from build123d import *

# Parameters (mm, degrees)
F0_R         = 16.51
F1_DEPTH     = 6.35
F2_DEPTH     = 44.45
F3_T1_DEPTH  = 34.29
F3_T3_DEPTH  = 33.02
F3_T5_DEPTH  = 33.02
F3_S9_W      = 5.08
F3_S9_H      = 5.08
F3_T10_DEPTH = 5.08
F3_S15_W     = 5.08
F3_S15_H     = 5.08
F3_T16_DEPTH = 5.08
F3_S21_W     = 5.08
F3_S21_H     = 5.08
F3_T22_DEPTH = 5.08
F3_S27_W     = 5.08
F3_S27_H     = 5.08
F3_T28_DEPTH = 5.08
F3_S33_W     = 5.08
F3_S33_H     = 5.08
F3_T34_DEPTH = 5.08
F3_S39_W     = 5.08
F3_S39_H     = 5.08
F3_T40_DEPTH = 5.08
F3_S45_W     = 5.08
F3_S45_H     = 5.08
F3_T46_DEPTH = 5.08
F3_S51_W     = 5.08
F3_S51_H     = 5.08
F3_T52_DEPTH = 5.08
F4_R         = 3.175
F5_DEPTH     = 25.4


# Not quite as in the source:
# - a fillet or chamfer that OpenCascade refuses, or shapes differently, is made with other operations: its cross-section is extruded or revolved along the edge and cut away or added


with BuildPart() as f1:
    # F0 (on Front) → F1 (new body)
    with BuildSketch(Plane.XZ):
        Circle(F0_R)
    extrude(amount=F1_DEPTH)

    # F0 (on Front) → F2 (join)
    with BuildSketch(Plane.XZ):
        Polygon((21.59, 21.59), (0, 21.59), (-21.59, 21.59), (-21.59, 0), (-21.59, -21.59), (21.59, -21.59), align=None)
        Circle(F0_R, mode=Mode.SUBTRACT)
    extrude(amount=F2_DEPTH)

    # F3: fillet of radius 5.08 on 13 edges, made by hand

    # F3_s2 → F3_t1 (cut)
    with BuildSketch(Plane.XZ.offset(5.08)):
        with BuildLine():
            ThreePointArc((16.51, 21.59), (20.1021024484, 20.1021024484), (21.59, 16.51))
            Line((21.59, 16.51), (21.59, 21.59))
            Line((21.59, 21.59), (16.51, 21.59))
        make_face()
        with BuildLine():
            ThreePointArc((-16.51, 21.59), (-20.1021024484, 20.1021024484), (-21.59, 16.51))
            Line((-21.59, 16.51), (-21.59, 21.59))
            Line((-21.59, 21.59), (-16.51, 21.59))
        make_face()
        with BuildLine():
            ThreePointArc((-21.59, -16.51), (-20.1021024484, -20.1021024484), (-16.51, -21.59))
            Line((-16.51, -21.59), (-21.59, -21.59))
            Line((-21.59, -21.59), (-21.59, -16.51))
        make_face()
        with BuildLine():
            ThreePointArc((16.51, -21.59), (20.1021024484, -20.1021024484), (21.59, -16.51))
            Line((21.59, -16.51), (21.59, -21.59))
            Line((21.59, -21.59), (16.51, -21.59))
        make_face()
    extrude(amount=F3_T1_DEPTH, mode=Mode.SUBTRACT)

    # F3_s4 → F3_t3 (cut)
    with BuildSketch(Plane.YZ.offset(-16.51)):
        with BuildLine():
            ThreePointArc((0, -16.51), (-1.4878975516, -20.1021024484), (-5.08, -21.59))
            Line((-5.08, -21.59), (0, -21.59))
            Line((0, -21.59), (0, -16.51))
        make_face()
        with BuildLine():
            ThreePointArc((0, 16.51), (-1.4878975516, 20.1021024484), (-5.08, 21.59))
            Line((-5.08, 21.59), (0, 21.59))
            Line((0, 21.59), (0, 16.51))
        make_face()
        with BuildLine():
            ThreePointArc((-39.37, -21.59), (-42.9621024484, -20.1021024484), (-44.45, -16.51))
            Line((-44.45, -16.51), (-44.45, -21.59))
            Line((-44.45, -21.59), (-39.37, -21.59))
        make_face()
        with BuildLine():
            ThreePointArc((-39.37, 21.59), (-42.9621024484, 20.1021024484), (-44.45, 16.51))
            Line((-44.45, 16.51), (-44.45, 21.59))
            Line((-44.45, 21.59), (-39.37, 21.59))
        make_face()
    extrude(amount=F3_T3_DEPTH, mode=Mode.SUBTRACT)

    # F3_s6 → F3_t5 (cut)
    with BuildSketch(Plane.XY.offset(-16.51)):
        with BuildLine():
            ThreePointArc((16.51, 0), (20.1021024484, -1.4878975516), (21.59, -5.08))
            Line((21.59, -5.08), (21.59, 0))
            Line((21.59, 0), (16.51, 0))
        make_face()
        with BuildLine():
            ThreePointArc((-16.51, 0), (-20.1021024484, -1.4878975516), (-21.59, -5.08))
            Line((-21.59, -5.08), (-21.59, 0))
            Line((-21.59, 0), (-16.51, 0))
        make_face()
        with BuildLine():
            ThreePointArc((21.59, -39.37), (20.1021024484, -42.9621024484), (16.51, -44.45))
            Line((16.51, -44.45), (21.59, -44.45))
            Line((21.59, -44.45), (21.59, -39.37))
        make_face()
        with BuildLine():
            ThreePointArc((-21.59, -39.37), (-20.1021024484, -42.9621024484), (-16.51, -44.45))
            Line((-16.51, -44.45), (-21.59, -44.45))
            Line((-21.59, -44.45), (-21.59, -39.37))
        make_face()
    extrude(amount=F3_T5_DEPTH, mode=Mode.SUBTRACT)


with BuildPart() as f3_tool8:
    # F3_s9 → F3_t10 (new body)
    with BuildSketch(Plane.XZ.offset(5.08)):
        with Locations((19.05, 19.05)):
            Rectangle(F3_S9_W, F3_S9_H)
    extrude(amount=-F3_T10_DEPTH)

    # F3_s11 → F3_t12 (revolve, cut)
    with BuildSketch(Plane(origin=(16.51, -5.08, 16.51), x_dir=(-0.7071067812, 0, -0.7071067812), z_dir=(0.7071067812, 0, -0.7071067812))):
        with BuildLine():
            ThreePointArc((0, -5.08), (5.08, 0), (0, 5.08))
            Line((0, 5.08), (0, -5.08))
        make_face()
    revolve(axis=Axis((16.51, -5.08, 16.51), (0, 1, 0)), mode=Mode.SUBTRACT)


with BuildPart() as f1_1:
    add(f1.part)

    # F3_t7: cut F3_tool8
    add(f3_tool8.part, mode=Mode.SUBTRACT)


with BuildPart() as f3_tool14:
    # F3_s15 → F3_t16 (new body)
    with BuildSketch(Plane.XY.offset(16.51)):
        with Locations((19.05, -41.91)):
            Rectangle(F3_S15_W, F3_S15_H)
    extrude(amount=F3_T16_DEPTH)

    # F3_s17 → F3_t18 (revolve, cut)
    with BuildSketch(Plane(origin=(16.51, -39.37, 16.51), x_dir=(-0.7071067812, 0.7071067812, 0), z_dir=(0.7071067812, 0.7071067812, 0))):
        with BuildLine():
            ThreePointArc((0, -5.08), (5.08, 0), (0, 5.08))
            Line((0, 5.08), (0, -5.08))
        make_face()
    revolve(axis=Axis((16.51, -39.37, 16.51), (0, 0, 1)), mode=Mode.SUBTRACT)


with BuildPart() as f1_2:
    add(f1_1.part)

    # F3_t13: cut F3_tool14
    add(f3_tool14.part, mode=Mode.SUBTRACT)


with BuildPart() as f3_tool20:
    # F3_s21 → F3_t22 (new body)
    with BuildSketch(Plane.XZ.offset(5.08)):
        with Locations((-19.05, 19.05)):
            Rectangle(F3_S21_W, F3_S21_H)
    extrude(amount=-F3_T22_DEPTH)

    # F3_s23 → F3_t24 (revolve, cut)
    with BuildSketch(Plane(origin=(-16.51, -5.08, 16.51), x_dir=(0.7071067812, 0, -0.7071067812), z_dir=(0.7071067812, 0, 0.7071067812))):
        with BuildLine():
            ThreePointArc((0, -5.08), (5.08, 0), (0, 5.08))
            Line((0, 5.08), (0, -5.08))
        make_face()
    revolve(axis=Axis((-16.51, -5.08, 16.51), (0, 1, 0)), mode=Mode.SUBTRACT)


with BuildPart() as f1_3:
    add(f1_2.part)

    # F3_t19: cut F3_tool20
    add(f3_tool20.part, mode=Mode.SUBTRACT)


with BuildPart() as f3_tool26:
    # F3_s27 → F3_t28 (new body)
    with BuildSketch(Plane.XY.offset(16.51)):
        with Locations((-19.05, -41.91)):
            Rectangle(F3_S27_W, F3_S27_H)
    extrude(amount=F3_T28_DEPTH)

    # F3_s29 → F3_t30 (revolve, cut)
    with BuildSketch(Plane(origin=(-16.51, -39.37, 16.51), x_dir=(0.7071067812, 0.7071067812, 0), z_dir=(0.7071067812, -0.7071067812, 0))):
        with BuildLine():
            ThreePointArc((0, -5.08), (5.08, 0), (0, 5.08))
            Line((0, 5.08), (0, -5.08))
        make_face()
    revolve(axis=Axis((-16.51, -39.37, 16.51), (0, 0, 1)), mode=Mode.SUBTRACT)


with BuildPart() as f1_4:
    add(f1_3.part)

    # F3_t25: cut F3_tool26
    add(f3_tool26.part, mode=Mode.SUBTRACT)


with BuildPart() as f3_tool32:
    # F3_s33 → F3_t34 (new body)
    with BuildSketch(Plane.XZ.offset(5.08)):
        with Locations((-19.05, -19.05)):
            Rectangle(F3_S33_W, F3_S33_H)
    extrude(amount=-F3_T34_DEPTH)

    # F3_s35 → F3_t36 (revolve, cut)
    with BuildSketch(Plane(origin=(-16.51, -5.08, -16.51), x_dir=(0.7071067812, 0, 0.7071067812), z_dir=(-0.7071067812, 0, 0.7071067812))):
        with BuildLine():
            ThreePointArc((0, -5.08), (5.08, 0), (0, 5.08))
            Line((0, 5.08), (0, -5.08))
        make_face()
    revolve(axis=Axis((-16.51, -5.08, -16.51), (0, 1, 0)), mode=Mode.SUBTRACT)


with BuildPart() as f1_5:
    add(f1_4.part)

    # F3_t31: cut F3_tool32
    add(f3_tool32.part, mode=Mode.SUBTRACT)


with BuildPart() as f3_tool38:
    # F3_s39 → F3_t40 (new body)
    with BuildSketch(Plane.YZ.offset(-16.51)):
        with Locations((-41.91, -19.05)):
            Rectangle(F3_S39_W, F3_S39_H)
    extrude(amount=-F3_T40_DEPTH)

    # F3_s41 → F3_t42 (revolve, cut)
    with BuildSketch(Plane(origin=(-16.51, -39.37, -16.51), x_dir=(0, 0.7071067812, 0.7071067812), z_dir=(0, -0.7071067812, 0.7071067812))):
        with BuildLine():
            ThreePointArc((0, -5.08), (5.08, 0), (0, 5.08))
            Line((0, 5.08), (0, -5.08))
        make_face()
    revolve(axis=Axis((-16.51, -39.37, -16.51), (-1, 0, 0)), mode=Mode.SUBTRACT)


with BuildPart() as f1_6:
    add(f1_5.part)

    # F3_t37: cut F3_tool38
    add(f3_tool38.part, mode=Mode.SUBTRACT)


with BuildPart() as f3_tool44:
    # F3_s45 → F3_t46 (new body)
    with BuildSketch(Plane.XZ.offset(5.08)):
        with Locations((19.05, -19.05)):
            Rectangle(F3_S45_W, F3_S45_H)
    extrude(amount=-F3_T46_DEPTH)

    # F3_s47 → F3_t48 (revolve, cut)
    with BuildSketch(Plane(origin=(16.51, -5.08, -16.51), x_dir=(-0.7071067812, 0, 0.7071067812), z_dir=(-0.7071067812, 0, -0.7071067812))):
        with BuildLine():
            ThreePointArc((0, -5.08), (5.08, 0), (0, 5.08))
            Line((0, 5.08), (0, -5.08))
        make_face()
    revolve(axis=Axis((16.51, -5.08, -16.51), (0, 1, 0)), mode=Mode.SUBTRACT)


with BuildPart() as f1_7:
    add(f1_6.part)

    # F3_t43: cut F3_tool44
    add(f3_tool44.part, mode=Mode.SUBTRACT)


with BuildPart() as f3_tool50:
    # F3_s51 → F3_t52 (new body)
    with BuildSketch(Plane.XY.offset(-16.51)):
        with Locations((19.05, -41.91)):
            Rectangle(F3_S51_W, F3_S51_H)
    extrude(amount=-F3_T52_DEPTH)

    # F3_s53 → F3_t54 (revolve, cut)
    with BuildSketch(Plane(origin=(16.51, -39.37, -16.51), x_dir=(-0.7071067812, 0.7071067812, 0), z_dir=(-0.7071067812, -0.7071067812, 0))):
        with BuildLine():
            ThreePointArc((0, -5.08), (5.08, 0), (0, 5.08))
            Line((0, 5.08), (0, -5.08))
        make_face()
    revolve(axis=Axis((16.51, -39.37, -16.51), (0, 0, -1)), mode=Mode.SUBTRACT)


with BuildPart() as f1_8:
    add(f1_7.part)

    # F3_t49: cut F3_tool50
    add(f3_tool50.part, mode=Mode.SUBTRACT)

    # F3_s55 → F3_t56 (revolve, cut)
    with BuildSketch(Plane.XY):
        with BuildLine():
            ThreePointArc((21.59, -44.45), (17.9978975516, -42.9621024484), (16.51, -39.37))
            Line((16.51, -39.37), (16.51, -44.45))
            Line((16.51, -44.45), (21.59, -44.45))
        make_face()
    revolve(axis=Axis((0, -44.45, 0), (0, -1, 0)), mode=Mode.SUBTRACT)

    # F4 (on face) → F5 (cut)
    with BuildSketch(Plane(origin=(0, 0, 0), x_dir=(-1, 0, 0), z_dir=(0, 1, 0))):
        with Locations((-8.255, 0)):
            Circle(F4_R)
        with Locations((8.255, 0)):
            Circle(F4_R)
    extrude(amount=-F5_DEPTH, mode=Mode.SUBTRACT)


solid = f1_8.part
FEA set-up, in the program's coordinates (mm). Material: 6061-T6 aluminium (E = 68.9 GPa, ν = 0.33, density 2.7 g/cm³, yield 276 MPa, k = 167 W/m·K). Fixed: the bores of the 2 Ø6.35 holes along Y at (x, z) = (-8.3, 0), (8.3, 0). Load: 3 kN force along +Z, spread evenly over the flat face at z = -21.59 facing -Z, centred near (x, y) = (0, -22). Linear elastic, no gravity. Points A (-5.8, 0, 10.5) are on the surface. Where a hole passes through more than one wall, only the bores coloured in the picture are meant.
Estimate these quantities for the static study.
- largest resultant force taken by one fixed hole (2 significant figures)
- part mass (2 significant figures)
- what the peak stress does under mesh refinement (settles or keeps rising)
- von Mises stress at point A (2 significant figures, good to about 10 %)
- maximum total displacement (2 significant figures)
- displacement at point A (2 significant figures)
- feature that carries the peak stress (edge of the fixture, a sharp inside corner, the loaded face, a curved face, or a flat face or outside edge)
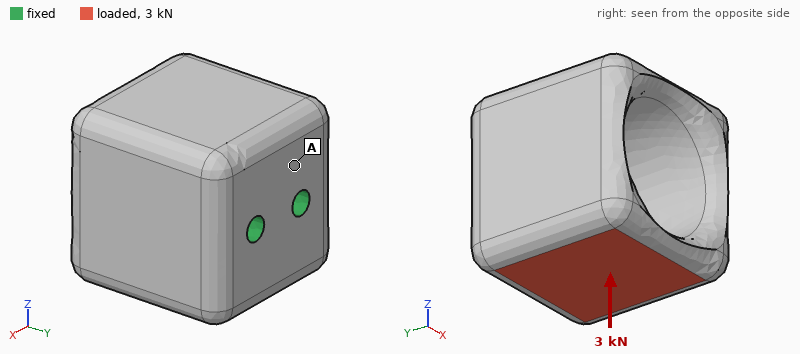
1.5 kN
130 g
keeps rising
27 MPa
0.13 mm
0.020 mm
edge of the fixture
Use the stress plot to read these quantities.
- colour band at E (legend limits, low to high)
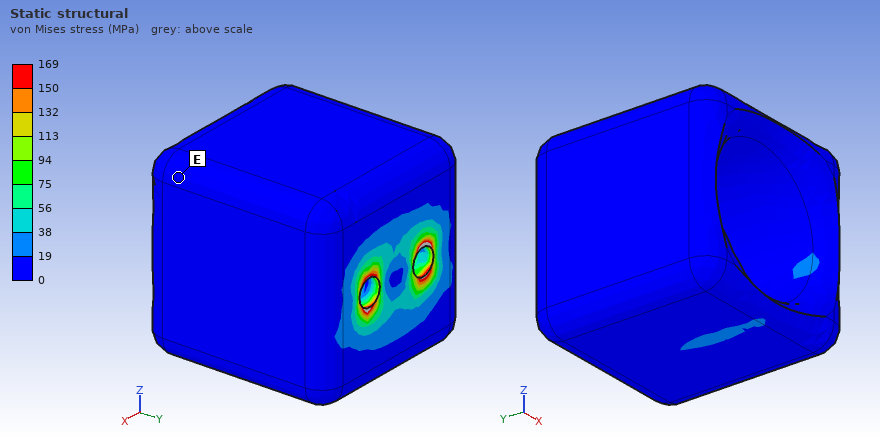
0 to 19 MPa
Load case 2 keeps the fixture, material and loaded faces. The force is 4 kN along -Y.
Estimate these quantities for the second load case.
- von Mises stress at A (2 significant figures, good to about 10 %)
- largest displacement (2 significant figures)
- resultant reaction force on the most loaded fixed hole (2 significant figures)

34 MPa
0.17 mm
2.0 kN
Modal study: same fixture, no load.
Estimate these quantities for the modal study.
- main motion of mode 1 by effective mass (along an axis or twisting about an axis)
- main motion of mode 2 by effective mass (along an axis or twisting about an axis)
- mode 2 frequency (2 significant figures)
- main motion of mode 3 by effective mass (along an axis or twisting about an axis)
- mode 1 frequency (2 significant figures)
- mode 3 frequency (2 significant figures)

along Z
along X
4300 Hz
twisting about Y
2700 Hz
8200 Hz
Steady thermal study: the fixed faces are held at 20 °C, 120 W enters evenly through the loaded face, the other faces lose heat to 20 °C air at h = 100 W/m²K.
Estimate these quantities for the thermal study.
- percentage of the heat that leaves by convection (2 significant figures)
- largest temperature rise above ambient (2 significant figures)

19 %
40 K
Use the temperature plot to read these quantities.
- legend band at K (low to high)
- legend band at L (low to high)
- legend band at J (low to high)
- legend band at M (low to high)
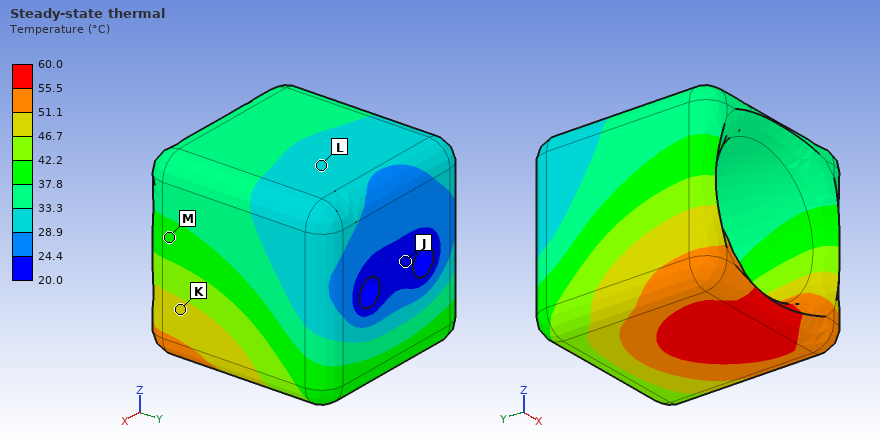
46.7 to 51.1 °C
28.9 to 33.3 °C
20.0 to 24.4 °C
37.8 to 42.2 °C
